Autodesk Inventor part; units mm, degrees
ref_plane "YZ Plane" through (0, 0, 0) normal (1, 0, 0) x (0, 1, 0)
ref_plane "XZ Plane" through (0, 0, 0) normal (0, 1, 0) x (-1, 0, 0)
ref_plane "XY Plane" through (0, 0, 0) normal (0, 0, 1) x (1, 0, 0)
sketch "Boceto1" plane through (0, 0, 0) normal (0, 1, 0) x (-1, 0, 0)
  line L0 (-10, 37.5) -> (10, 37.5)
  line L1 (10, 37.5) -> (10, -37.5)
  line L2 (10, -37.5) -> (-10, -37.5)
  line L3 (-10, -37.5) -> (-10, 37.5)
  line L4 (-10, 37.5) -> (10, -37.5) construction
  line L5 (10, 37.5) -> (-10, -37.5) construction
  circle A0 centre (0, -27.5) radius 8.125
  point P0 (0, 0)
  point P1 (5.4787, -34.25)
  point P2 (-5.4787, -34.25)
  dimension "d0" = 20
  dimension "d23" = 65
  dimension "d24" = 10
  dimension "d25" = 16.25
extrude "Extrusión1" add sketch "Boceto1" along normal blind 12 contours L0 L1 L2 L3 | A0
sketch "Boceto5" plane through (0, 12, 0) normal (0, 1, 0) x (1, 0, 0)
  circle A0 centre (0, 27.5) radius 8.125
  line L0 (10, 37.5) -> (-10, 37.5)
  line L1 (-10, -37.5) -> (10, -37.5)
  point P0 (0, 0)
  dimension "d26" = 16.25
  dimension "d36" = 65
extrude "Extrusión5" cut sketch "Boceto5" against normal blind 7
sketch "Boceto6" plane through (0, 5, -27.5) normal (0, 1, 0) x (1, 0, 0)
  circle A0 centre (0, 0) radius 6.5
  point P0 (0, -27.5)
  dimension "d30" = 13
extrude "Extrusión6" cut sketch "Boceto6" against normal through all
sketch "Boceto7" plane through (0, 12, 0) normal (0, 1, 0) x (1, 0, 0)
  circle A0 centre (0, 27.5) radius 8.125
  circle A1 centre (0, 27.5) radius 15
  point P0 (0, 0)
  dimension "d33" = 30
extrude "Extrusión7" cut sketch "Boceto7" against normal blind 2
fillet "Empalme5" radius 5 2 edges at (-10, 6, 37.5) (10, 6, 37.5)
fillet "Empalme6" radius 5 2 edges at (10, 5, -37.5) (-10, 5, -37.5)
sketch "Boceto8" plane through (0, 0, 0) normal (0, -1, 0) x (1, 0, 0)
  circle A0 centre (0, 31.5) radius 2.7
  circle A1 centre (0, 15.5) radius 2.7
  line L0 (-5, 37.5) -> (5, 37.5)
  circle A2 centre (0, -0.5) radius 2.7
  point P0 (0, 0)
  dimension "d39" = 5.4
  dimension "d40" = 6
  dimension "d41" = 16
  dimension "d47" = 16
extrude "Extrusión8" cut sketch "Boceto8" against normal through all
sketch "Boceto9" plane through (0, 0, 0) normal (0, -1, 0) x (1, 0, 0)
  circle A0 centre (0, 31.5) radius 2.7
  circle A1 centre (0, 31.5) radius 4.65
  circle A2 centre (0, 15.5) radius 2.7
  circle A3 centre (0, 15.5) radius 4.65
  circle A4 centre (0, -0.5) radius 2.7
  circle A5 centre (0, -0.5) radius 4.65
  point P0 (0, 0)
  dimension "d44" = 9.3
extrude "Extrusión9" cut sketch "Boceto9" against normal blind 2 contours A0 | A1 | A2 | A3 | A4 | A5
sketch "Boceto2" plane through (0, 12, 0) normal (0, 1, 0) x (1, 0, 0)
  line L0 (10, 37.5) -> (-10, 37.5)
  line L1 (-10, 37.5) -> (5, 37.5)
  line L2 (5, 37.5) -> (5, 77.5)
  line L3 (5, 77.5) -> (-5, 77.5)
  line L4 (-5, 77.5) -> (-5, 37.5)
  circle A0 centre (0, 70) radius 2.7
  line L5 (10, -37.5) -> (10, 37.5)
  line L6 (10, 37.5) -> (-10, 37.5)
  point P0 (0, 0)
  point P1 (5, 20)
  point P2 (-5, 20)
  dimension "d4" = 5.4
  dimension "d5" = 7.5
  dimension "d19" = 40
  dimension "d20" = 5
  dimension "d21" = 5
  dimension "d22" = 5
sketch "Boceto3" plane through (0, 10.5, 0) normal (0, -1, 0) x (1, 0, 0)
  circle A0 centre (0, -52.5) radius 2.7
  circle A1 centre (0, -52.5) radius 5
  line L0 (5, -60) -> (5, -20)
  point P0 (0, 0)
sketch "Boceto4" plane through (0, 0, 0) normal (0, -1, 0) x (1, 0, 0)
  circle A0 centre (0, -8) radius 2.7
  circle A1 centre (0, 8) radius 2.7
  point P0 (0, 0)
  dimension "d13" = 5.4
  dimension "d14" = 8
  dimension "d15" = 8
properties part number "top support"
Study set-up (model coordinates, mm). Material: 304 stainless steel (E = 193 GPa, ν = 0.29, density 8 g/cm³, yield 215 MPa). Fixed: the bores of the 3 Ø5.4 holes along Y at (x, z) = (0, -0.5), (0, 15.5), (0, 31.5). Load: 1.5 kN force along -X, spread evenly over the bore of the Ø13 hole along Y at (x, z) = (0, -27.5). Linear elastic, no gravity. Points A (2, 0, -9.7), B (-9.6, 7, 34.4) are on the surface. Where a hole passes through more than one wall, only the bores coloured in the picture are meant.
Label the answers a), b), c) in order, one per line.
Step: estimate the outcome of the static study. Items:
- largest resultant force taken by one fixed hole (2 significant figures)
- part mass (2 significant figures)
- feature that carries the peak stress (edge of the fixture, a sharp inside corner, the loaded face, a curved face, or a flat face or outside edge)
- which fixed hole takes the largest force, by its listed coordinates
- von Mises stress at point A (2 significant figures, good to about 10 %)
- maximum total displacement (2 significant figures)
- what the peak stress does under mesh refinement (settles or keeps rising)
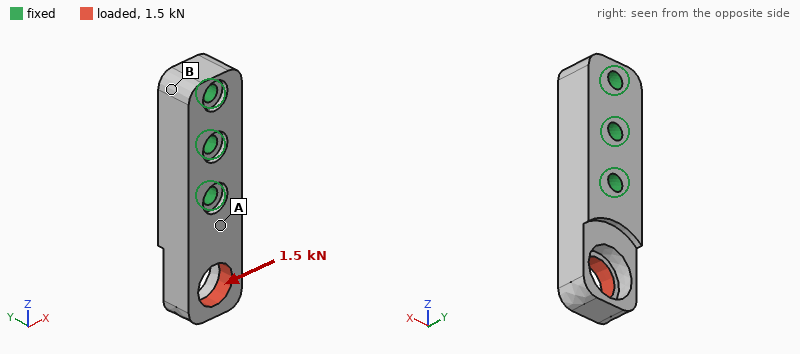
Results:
a) 2.8 kN
b) 110 g
c) edge of the fixture
d) (0, -0.5)
e) 25 MPa
f) 33 µm
g) keeps rising
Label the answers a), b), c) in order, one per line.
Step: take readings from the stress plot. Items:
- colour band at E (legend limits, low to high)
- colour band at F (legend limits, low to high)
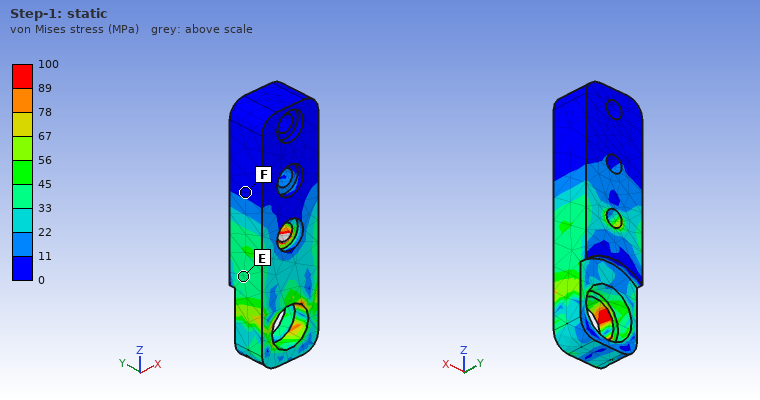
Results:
a) 33 to 45 MPa
b) 0 to 11 MPa
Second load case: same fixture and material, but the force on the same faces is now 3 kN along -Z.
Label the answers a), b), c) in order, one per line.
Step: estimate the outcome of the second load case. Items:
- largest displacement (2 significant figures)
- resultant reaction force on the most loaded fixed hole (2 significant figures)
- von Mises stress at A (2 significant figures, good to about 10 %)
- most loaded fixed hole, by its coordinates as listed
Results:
a) 22 µm
b) 2.4 kN
c) 27 MPa
d) (0, -0.5)
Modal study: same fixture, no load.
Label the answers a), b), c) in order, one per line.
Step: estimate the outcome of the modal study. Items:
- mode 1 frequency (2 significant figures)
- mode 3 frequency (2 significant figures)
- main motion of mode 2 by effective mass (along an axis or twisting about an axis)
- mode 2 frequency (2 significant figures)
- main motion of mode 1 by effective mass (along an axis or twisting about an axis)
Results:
a) 7500 Hz
b) 15 kHz
c) along X
d) 8900 Hz
e) along Y
